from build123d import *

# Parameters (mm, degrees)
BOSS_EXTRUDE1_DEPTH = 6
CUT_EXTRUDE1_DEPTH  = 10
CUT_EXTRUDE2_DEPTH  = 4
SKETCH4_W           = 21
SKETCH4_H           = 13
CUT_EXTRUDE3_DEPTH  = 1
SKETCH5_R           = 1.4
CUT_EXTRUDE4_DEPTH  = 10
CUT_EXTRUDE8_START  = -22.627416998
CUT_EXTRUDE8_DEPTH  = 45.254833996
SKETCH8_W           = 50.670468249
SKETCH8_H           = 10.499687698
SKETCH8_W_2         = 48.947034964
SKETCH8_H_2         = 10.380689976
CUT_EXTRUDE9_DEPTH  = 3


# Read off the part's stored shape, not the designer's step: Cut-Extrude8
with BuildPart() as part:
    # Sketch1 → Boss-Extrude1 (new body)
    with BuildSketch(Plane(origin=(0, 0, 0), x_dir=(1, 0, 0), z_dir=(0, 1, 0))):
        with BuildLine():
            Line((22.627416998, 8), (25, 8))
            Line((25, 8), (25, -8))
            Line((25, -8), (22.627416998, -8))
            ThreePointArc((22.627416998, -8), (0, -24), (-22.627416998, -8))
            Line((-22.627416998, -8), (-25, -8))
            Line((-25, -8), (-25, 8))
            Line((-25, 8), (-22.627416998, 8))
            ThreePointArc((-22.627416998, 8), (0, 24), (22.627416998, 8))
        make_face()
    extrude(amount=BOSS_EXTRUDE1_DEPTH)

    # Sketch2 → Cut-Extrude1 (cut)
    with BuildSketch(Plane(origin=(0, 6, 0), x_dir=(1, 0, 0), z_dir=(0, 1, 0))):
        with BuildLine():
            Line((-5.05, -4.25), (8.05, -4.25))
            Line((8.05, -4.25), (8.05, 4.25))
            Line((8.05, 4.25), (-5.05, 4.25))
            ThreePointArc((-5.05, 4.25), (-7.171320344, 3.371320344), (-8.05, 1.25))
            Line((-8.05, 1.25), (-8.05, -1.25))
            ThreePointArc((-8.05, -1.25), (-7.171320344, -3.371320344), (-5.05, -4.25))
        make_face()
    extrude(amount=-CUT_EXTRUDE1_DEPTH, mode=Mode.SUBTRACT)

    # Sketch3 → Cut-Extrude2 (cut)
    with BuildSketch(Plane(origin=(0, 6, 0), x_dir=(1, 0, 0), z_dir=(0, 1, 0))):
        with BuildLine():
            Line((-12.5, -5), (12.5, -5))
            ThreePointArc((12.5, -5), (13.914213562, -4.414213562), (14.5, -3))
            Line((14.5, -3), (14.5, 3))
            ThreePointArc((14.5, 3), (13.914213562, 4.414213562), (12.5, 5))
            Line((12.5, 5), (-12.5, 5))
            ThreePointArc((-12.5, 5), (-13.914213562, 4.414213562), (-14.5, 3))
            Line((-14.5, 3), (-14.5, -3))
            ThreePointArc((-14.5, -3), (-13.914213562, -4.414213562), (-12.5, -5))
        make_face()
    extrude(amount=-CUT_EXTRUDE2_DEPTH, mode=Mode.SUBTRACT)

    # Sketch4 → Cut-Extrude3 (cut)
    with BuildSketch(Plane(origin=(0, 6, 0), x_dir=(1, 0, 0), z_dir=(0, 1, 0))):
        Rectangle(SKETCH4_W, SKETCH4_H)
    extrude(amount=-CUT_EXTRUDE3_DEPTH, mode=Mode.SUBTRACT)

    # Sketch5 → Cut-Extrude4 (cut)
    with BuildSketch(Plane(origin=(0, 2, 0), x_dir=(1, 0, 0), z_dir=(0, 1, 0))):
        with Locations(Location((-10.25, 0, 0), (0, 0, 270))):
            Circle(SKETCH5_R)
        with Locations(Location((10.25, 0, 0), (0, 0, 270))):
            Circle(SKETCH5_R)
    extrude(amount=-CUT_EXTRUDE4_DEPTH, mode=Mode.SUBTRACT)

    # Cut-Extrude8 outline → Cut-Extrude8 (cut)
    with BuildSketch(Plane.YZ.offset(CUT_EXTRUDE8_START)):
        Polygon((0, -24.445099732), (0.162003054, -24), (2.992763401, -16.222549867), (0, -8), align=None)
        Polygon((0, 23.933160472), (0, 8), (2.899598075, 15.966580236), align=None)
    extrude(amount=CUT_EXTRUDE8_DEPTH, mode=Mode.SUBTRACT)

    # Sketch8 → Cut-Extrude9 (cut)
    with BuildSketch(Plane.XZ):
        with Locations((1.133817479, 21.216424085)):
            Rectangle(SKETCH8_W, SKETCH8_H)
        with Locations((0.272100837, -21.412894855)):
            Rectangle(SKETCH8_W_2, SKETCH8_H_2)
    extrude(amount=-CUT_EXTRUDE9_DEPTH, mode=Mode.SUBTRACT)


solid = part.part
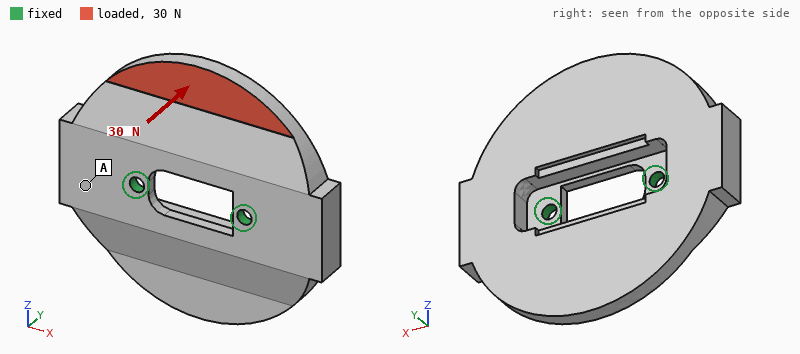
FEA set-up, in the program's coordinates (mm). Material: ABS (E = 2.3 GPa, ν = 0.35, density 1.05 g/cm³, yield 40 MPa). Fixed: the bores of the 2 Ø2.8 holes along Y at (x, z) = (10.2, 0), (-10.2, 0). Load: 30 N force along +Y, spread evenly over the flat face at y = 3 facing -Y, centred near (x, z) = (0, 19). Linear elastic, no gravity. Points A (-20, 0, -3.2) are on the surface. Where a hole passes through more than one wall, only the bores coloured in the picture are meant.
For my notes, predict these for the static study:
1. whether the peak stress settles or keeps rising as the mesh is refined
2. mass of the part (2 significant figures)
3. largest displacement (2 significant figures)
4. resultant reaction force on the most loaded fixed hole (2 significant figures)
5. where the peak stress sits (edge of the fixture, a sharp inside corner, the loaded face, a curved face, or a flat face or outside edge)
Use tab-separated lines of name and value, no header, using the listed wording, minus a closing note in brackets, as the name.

whether the peak stress settles or keeps rising as the mesh is refined	keeps rising
mass of the part	7.9 g
largest displacement	0.69 mm
resultant reaction force on the most loaded fixed hole	15 N
where the peak stress sits	edge of the fixture
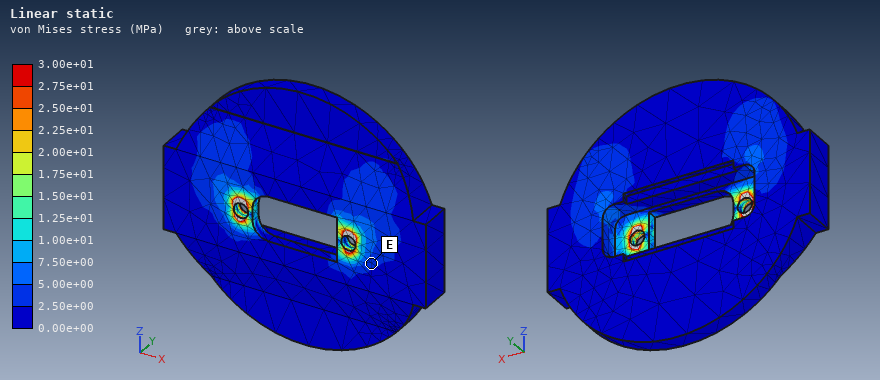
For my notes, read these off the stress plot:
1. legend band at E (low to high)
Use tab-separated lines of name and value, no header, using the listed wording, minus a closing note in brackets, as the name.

legend band at E	2.50e+00 to 5.00e+00 MPa
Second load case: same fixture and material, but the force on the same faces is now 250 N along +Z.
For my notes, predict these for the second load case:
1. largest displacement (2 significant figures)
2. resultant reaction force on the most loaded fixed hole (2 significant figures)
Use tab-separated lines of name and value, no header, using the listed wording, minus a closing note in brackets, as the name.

largest displacement	0.49 mm
resultant reaction force on the most loaded fixed hole	130 N
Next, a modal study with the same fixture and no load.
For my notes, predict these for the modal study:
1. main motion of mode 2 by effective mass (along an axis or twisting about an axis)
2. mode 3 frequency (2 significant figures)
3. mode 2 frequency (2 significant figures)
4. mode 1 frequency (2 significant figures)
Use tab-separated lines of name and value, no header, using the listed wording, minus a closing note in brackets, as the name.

main motion of mode 2 by effective mass	along Y
mode 3 frequency	2400 Hz
mode 2 frequency	2200 Hz
mode 1 frequency	800 Hz
